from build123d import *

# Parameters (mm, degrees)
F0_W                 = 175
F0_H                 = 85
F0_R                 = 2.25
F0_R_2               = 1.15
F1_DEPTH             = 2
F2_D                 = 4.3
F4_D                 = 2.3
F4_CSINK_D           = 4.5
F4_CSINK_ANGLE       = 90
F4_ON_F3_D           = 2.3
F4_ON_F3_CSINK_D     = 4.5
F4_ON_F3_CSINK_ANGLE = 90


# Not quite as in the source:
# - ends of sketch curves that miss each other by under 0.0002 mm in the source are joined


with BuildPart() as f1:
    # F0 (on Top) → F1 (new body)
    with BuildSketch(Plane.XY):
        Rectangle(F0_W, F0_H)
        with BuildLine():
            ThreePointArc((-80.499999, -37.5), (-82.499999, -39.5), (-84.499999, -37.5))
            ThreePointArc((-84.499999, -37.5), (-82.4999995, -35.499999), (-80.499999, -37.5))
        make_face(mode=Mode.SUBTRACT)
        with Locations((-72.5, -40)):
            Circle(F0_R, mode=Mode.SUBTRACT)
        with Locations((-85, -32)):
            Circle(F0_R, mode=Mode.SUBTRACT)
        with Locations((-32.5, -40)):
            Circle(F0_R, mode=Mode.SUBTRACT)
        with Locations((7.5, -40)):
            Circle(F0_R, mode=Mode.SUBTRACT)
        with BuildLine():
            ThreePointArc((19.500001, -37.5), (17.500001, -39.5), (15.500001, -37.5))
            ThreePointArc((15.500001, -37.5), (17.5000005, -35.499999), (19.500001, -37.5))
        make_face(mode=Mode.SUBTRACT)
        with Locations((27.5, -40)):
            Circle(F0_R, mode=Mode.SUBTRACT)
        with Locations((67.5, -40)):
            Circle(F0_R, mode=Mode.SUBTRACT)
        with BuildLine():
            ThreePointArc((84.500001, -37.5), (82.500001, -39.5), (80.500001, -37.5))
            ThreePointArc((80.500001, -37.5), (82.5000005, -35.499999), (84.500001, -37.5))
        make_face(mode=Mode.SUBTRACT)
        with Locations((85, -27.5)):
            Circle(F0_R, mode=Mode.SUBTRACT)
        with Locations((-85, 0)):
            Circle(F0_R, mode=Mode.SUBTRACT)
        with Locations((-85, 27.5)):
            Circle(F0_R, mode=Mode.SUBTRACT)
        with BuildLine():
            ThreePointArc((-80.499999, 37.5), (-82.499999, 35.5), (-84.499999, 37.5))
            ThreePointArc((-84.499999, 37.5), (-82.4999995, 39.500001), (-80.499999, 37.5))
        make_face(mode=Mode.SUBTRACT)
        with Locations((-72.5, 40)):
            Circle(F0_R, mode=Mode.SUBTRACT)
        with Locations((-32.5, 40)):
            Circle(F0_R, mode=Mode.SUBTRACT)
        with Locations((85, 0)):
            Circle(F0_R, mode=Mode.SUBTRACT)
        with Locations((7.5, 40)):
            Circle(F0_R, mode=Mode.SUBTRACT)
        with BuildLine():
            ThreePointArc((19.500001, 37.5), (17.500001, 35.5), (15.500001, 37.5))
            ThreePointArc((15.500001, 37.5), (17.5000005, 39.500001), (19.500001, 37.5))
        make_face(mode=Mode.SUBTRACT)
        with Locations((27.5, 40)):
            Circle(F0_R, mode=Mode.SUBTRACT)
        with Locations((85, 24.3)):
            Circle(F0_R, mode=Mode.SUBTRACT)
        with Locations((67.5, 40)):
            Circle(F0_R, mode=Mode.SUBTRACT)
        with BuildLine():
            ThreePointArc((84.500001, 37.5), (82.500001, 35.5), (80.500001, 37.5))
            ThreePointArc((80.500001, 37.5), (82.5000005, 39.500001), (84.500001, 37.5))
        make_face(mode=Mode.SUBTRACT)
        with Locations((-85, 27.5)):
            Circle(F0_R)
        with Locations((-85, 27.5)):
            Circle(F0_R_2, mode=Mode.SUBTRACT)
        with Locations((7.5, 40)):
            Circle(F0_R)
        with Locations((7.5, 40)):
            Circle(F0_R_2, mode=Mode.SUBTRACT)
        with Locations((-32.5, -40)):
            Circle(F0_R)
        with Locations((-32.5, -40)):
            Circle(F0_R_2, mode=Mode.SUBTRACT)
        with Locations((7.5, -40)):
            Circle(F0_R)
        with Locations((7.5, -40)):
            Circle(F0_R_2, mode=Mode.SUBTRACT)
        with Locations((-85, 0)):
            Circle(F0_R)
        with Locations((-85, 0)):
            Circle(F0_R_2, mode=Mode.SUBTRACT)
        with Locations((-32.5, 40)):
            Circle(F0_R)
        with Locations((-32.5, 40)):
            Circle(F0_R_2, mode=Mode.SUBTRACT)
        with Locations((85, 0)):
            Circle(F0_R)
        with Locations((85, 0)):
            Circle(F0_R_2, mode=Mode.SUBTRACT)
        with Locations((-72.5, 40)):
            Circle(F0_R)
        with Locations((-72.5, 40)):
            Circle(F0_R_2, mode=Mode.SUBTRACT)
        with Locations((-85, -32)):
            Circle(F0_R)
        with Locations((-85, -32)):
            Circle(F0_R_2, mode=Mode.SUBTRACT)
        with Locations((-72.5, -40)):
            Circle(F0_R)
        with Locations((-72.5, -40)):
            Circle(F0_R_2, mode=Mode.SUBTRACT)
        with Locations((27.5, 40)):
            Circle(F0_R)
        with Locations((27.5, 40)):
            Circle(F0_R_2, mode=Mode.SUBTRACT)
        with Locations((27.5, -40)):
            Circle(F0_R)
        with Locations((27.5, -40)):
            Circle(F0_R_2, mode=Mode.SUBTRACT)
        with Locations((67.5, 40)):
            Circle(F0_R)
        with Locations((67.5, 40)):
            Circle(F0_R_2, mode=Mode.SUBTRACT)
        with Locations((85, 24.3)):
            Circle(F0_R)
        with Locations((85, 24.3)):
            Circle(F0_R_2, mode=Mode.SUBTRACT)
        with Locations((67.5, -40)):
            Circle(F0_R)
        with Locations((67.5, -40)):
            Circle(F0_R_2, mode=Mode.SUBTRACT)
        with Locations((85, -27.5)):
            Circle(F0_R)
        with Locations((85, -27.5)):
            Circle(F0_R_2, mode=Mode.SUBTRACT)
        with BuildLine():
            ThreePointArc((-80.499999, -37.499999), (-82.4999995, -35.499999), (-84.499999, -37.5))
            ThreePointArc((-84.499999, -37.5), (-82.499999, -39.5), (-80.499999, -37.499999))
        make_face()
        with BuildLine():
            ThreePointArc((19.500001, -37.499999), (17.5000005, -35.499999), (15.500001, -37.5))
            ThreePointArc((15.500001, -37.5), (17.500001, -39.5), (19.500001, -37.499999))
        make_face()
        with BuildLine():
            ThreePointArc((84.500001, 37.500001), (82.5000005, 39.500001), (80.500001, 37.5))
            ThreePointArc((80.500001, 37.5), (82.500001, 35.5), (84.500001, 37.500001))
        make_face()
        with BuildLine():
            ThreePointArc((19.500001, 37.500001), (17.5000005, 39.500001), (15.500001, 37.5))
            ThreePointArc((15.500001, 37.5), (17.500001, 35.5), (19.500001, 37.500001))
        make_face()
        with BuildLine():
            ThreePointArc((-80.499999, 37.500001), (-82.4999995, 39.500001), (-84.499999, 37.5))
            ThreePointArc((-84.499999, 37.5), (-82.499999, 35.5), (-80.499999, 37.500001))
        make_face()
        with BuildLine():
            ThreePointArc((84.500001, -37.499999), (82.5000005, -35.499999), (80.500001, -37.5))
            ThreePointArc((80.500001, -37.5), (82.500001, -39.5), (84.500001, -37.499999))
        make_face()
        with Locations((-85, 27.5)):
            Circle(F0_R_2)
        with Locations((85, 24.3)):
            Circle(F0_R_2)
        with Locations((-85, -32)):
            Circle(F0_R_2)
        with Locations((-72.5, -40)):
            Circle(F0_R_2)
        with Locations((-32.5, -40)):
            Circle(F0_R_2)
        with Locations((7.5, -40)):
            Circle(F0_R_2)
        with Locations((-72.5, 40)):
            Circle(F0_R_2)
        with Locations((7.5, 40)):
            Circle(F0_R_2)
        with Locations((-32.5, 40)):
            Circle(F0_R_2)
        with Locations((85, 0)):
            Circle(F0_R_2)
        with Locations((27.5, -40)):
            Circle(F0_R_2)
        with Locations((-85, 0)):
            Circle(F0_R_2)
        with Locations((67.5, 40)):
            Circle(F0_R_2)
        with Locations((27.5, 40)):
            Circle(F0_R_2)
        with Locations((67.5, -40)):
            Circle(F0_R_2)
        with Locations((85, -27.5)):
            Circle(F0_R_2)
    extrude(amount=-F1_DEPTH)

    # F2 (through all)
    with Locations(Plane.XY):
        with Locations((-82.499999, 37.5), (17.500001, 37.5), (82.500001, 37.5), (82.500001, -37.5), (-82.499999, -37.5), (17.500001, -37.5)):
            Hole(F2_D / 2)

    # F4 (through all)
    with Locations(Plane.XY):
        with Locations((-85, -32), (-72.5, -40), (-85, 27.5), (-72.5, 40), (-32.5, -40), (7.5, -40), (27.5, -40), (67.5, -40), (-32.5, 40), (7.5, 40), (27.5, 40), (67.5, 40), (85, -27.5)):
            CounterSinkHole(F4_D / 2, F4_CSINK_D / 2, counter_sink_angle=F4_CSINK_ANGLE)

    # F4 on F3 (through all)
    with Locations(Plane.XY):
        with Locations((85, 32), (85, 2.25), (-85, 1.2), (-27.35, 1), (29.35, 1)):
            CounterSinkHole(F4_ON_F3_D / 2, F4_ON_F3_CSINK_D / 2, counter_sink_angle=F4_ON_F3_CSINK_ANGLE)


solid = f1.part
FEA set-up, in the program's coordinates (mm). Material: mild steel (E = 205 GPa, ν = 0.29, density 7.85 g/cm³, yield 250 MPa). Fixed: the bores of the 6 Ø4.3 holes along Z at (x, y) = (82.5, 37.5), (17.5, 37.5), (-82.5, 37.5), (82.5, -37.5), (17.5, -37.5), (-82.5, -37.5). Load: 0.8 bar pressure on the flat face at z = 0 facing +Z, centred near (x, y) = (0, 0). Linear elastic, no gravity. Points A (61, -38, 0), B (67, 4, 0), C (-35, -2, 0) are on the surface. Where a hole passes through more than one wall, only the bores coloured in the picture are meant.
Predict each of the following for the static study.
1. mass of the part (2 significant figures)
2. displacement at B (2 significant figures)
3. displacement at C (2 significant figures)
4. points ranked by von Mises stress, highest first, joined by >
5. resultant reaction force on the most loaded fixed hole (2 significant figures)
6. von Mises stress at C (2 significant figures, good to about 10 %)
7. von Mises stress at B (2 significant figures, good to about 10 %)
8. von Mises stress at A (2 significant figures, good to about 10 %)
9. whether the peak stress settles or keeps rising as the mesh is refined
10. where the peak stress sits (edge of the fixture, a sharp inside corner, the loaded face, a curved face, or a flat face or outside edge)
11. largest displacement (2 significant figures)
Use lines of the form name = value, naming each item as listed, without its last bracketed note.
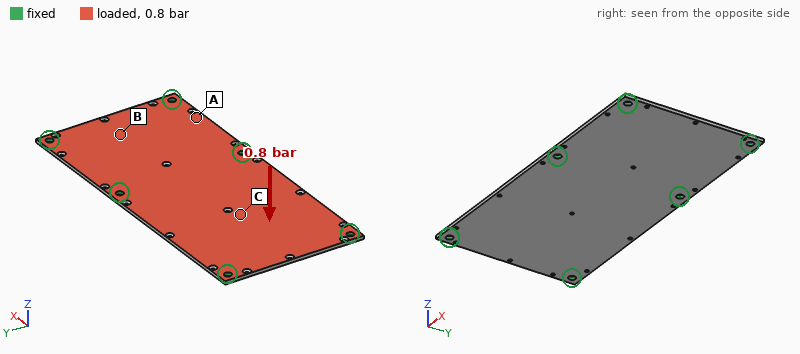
mass of the part = 230 g
displacement at B = 0.077 mm
displacement at C = 0.26 mm
points ranked by von Mises stress, highest first, joined by > = C > B > A
resultant reaction force on the most loaded fixed hole = 290 N
von Mises stress at C = 51 MPa
von Mises stress at B = 29 MPa
von Mises stress at A = 18 MPa
whether the peak stress settles or keeps rising as the mesh is refined = keeps rising
where the peak stress sits = edge of the fixture
largest displacement = 0.26 mm
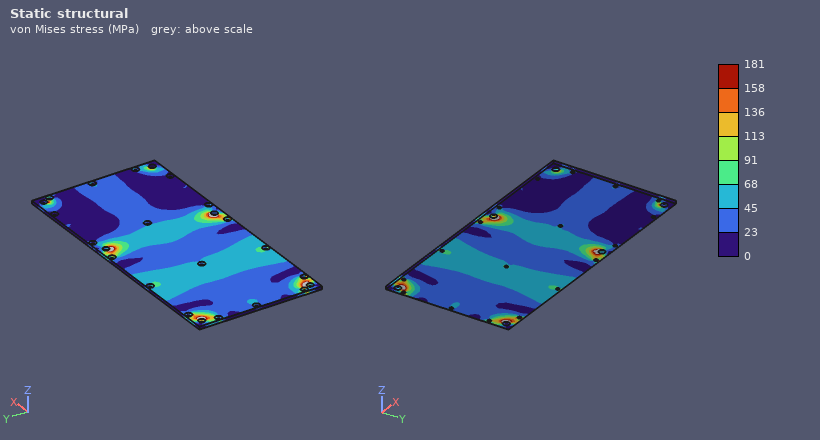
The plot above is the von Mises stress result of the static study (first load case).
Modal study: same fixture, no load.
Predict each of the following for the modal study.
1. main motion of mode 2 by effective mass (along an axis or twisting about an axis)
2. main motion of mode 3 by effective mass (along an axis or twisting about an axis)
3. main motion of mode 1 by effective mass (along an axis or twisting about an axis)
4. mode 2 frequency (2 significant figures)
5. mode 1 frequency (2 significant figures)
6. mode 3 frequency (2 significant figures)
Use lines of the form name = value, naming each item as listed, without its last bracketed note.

main motion of mode 2 by effective mass = twisting about X
main motion of mode 3 by effective mass = along Z
main motion of mode 1 by effective mass = along Z
mode 2 frequency = 1300 Hz
mode 1 frequency = 820 Hz
mode 3 frequency = 1400 Hz
